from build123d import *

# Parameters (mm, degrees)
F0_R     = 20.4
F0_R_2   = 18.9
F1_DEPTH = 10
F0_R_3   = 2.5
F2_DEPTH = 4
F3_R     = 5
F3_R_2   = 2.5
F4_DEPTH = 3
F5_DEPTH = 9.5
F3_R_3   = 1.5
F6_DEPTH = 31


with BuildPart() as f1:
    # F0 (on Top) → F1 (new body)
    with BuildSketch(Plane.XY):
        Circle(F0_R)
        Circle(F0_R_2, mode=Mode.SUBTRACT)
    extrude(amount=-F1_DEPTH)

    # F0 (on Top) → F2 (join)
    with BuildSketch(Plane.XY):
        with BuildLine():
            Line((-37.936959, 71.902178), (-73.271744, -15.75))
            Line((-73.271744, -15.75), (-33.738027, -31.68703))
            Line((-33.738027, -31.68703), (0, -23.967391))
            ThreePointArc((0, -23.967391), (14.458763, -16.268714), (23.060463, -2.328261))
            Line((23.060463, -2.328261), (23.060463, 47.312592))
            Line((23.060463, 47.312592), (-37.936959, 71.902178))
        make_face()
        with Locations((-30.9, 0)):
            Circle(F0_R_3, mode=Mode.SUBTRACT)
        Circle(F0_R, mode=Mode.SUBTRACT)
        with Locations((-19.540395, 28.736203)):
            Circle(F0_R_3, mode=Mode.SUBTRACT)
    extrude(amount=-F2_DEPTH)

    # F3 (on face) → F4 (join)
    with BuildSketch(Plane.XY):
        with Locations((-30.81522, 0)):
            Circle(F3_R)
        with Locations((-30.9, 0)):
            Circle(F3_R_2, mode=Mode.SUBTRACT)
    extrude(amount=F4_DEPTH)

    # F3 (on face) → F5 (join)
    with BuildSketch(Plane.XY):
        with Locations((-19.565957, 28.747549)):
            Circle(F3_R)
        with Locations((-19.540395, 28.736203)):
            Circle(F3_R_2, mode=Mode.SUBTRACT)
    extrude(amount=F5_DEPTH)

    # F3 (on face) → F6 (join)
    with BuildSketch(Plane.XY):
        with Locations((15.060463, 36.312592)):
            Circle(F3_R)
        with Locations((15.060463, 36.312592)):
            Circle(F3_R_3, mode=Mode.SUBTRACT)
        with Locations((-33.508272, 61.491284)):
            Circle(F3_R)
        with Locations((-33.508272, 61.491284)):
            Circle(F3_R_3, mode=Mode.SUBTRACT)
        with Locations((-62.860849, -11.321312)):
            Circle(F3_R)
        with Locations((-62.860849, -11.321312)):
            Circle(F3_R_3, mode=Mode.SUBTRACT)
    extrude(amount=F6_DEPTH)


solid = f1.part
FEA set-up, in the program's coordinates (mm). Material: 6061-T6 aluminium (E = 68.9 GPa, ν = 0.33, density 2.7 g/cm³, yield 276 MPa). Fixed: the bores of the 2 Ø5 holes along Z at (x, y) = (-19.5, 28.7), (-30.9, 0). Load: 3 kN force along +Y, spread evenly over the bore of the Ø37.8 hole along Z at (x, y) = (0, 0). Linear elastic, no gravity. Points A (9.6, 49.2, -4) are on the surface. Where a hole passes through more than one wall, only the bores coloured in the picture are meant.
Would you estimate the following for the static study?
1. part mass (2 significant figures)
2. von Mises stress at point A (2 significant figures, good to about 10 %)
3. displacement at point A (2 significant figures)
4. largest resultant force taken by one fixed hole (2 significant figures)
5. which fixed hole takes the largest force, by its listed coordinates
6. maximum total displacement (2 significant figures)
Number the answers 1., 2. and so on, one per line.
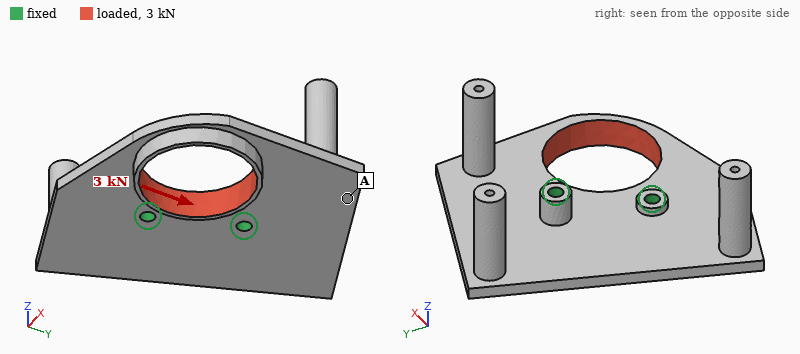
1. 85 g
2. 18 MPa
3. 0.060 mm
4. 3.0 kN
5. (-19.5, 28.7)
6. 0.23 mm
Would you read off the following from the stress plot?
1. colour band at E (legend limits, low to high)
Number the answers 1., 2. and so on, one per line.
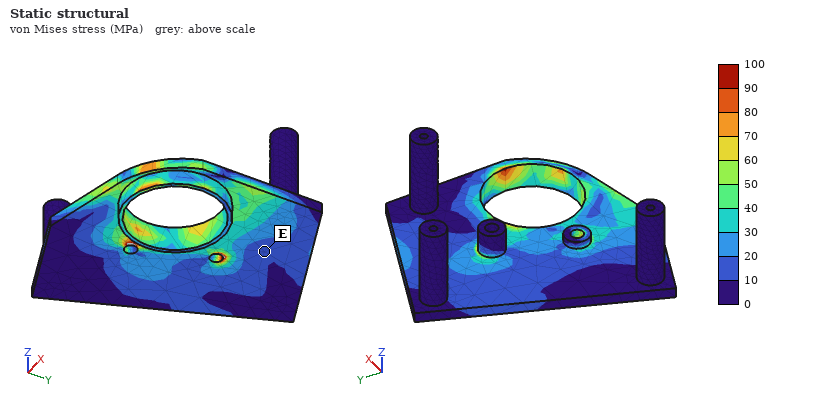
1. 10 to 20 MPa
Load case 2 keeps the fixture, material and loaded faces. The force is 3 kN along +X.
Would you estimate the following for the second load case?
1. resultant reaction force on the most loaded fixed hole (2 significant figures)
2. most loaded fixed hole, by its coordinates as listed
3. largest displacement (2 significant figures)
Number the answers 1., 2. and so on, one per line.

1. 2.8 kN
2. (-30.9, 0)
3. 0.35 mm
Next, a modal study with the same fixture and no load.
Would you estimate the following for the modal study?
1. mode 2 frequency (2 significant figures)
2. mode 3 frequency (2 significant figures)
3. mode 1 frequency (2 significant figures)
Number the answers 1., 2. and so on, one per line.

1. 1500 Hz
2. 1500 Hz
3. 1300 Hz
